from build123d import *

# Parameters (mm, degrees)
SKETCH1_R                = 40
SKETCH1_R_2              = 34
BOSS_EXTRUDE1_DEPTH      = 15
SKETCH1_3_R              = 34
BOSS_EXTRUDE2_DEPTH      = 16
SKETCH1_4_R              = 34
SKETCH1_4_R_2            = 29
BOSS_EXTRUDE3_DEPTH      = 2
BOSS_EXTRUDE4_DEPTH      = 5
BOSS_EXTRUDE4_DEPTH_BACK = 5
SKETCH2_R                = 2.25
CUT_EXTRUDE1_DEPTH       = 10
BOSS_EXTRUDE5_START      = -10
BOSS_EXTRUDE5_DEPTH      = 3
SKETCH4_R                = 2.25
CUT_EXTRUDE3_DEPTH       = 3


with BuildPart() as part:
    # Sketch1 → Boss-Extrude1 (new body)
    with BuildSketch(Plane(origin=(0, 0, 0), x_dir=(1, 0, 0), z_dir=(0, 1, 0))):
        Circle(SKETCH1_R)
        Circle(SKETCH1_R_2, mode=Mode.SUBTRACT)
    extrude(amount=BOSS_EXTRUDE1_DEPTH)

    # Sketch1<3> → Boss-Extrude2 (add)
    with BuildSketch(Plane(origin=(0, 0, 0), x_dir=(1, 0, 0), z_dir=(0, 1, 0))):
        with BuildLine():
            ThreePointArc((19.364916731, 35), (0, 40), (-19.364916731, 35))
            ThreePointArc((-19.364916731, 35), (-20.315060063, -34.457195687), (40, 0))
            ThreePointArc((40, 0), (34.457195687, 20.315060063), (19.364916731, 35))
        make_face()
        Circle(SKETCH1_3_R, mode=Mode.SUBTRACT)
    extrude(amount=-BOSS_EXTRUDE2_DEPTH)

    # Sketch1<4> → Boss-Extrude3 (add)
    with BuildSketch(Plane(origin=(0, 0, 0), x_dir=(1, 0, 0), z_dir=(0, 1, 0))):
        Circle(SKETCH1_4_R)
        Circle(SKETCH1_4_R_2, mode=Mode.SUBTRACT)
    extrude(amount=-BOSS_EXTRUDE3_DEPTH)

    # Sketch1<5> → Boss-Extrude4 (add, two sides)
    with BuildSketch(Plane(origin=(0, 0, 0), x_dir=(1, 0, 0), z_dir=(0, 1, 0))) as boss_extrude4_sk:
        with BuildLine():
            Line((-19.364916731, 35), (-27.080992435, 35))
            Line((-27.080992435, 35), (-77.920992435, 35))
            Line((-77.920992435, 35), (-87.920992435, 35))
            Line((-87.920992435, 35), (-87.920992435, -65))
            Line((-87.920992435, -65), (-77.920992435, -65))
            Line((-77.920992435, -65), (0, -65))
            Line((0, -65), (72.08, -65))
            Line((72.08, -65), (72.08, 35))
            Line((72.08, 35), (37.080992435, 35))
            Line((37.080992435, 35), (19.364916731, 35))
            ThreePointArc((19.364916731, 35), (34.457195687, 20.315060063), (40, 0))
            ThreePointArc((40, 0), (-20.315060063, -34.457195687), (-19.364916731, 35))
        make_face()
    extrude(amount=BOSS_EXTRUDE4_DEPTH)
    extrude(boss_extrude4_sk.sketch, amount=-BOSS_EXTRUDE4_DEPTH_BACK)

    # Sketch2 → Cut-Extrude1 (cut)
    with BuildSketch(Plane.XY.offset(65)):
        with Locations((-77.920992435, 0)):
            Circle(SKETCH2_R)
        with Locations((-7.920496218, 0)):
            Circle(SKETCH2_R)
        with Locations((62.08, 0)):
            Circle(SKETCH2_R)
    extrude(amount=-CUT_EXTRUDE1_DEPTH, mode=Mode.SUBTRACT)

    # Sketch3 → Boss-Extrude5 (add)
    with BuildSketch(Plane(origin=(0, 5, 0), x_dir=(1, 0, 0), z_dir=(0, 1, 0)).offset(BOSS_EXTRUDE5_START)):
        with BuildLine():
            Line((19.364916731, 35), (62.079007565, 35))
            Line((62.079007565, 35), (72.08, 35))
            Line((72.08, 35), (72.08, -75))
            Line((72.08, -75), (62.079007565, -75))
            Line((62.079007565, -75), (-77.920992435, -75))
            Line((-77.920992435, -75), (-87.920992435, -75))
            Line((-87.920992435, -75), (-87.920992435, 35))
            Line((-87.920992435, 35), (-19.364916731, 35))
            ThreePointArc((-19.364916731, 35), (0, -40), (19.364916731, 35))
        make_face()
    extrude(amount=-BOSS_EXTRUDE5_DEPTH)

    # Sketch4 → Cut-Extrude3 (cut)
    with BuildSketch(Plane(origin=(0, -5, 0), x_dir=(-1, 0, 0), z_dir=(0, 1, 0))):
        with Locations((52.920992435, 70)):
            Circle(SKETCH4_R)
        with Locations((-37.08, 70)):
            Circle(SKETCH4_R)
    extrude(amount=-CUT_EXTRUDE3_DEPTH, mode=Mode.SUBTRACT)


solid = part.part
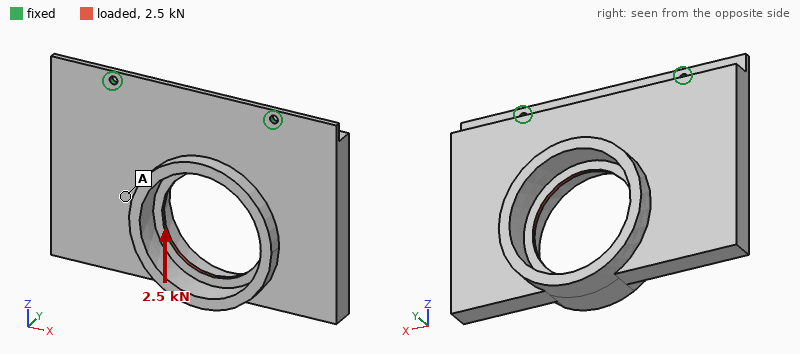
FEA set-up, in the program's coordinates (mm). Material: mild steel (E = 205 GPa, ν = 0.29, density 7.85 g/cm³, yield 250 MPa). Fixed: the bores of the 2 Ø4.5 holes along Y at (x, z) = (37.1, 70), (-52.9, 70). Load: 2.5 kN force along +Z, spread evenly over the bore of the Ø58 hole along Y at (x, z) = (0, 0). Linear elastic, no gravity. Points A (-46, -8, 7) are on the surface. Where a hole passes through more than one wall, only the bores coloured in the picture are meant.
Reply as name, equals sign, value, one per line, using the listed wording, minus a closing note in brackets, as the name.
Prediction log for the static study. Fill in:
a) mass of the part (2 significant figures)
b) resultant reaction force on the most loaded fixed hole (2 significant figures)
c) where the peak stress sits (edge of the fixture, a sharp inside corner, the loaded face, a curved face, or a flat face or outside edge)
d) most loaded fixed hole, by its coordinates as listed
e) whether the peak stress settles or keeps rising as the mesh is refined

mass of the part = 1.5 kg
resultant reaction force on the most loaded fixed hole = 1.5 kN
where the peak stress sits = edge of the fixture
most loaded fixed hole, by its coordinates as listed = (37.1, 70)
whether the peak stress settles or keeps rising as the mesh is refined = keeps rising
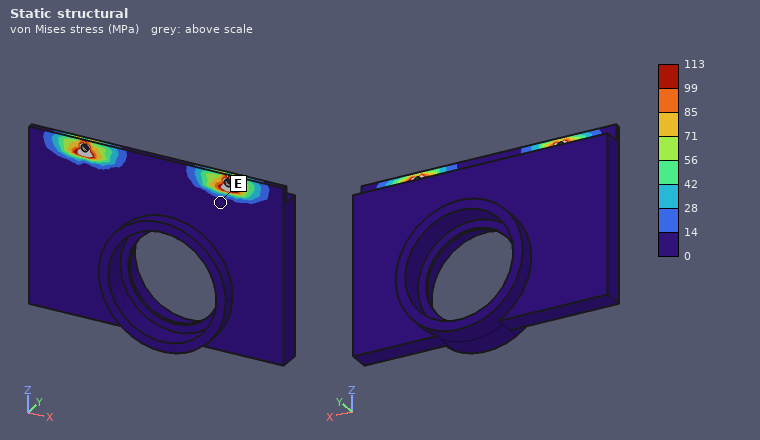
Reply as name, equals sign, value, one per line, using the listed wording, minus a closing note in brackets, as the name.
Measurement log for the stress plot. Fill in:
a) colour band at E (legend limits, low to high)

colour band at E = 0 to 14 MPa
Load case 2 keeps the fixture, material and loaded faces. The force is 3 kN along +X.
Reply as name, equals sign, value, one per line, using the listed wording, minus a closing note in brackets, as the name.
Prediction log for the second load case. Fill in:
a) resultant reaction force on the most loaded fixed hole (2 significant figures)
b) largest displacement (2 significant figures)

resultant reaction force on the most loaded fixed hole = 2.8 kN
largest displacement = 25 µm
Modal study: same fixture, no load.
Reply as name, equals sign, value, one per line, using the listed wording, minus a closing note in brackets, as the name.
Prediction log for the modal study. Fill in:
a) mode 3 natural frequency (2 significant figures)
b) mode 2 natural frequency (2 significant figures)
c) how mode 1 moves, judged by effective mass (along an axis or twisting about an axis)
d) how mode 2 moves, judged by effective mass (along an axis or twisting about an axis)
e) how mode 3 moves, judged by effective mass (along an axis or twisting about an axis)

mode 3 natural frequency = 2200 Hz
mode 2 natural frequency = 950 Hz
how mode 1 moves, judged by effective mass = along Y
how mode 2 moves, judged by effective mass = twisting about Z
how mode 3 moves, judged by effective mass = along X
